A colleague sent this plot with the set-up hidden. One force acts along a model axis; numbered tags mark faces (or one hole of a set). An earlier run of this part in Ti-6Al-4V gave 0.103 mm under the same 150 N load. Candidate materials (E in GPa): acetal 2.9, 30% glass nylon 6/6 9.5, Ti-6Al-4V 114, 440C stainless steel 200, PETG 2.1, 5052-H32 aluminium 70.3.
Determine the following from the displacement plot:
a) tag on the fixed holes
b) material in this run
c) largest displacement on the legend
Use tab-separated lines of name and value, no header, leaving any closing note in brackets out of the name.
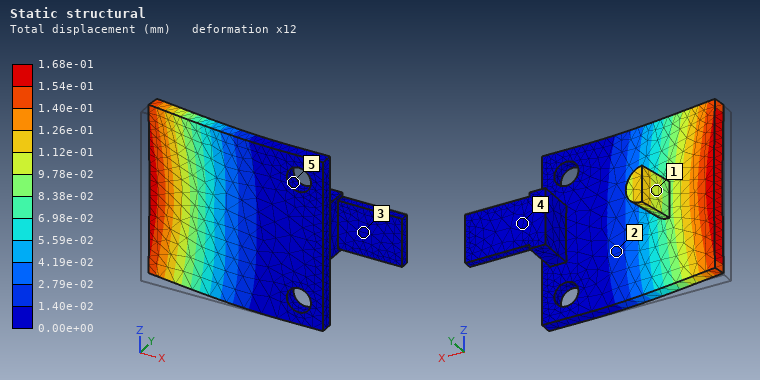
tag on the fixed holes	5
material in this run	5052-H32 aluminium
largest displacement on the legend	1.68e-01 mm
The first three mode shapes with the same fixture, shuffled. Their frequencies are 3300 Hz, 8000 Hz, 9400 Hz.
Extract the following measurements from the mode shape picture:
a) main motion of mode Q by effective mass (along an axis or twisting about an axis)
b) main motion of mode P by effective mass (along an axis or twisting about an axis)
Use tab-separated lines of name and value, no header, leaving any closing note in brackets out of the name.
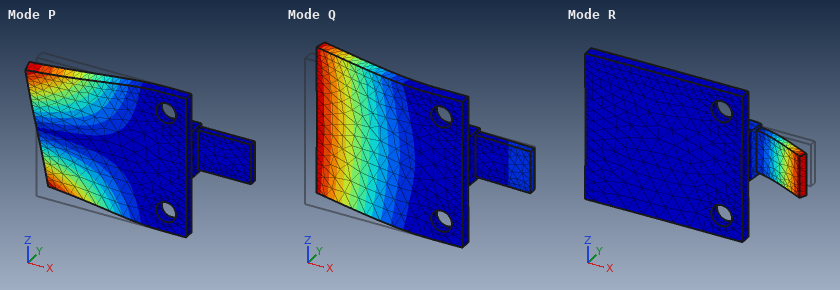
main motion of mode Q by effective mass	along Y
main motion of mode P by effective mass	twisting about X
